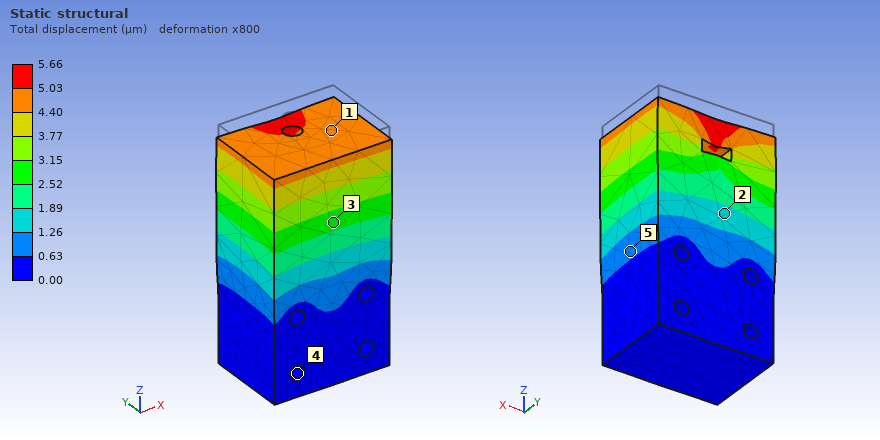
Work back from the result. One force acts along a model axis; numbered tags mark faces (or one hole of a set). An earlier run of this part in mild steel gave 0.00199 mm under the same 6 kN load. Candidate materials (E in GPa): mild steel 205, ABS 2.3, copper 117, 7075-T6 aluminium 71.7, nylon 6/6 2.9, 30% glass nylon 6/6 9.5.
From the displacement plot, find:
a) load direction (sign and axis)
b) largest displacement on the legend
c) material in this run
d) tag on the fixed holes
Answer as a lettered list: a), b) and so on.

a) -Z
b) 5.66 µm
c) 7075-T6 aluminium
d) 4
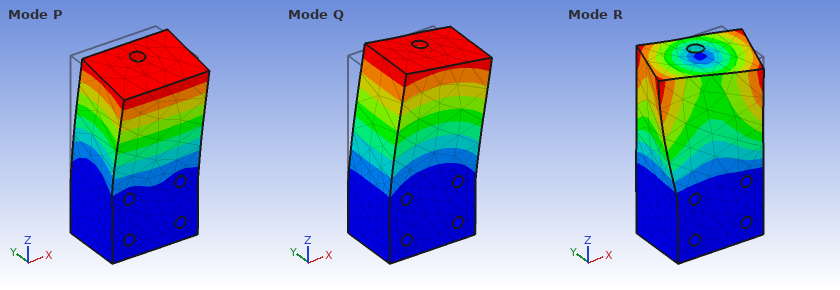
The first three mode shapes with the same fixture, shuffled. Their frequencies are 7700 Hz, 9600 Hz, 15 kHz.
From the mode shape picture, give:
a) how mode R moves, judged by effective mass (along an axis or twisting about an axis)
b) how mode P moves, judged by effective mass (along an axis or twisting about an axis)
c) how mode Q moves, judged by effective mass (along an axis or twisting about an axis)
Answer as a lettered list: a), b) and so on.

a) twisting about Z
b) along Y
c) along X
